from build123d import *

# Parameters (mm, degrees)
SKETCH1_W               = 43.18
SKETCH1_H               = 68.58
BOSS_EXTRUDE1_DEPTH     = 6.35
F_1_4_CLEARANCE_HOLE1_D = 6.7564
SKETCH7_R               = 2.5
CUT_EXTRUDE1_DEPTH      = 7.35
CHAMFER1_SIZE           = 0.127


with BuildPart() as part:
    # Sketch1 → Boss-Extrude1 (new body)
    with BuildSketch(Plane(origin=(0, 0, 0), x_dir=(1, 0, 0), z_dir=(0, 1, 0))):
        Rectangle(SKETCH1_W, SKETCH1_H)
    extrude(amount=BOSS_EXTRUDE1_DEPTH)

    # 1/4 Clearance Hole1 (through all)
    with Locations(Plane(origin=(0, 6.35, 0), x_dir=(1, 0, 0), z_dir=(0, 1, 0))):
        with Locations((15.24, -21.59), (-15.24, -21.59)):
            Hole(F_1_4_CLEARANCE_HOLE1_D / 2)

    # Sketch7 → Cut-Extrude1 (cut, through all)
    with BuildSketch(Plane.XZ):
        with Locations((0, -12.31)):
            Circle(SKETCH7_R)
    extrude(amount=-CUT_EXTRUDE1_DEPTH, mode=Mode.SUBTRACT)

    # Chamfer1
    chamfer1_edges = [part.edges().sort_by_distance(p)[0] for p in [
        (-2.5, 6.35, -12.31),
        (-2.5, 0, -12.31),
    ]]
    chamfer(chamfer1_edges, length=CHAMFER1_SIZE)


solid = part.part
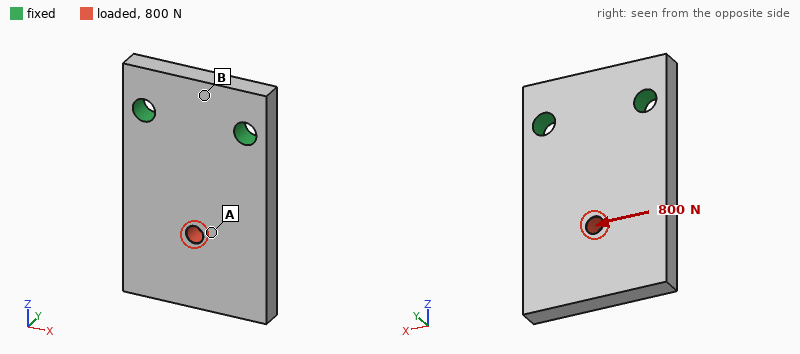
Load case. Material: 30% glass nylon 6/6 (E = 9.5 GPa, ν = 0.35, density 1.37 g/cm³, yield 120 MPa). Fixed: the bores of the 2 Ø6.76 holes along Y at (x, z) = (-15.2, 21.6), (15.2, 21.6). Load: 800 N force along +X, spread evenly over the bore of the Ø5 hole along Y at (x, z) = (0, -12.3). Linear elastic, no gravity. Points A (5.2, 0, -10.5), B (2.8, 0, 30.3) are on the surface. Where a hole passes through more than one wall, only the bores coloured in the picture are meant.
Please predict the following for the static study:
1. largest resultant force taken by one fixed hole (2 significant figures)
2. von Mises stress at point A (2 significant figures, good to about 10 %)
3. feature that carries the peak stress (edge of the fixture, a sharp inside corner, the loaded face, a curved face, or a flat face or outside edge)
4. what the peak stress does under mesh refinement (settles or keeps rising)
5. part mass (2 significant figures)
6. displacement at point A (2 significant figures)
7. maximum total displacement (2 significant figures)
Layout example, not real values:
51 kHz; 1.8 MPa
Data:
890 N; 7.7 MPa; edge of the fixture; keeps rising; 25 g; 52 µm; 82 µm
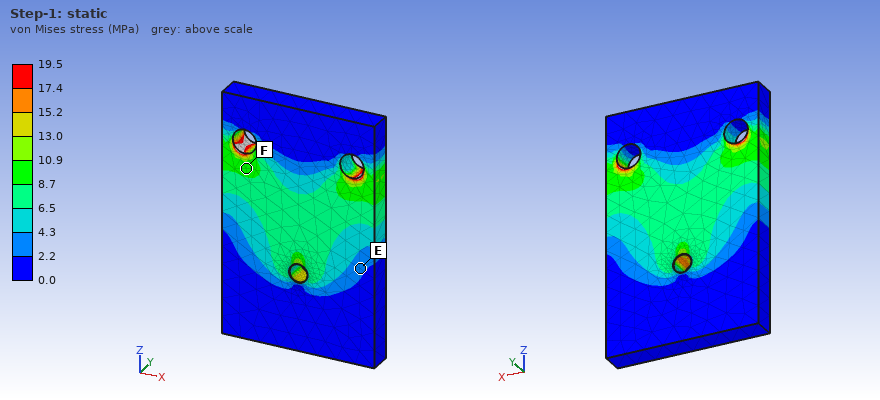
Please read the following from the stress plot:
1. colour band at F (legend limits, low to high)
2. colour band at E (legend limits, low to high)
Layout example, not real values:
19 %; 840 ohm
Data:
8.7 to 10.9 MPa; 2.2 to 4.3 MPa
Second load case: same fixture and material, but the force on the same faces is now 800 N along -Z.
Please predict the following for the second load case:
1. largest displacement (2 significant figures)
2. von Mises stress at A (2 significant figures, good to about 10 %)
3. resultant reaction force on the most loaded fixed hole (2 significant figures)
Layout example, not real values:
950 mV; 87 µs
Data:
18 µm; 4.1 MPa; 410 N
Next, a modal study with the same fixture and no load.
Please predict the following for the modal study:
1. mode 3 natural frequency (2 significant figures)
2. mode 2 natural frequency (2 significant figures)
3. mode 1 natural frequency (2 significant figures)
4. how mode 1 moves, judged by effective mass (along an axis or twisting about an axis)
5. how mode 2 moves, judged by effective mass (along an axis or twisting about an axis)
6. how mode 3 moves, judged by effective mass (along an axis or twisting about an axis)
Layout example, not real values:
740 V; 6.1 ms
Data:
4400 Hz; 2500 Hz; 890 Hz; along Y; twisting about Z; along X
